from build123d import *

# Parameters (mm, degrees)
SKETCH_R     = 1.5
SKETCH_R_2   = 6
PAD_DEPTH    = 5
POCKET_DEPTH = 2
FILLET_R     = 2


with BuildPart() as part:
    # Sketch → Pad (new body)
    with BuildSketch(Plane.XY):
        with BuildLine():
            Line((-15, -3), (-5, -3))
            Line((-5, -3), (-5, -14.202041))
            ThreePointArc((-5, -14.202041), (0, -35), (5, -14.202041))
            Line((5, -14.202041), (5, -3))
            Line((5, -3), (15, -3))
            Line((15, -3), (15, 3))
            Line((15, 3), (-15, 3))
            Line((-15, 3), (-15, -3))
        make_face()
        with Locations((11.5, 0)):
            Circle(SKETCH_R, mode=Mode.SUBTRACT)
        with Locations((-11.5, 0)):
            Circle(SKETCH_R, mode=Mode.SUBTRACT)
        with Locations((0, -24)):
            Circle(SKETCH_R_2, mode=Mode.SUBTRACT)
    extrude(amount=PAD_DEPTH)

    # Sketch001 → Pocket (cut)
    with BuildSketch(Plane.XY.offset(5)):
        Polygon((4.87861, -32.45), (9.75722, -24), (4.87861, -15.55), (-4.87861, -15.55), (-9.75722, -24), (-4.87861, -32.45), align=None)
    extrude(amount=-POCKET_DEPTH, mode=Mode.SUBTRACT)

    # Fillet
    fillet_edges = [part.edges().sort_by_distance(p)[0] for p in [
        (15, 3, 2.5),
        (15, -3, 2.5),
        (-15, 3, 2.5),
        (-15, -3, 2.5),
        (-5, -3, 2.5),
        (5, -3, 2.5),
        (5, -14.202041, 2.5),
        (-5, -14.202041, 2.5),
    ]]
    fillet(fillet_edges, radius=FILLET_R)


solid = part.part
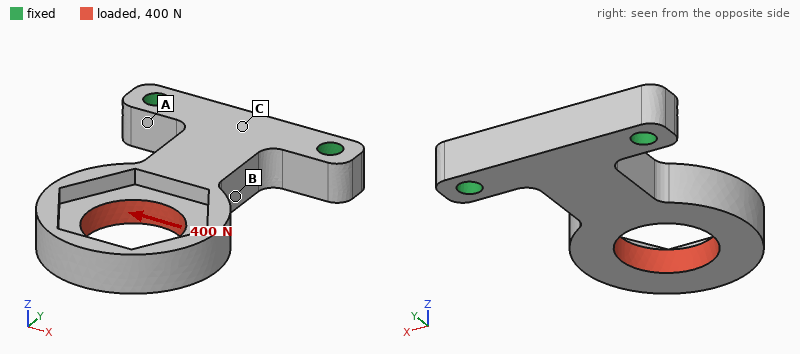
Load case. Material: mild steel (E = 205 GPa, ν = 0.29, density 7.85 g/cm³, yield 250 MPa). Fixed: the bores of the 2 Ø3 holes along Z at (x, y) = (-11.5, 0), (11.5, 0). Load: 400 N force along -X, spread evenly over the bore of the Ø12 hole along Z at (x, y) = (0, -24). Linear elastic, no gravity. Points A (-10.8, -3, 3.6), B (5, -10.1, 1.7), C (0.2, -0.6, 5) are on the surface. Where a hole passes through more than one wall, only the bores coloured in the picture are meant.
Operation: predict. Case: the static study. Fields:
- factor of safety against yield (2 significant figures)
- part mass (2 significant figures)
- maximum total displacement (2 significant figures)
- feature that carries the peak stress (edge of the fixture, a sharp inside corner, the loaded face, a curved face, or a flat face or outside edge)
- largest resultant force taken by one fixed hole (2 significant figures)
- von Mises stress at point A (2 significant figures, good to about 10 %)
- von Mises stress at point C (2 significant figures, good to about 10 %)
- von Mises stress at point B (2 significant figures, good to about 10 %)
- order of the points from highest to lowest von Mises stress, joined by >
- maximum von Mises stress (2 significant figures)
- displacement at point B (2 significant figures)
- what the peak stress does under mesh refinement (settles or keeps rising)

1.5
19 g
52 µm
a curved face
570 N
19 MPa
44 MPa
70 MPa
B > C > A
170 MPa
8.0 µm
settles
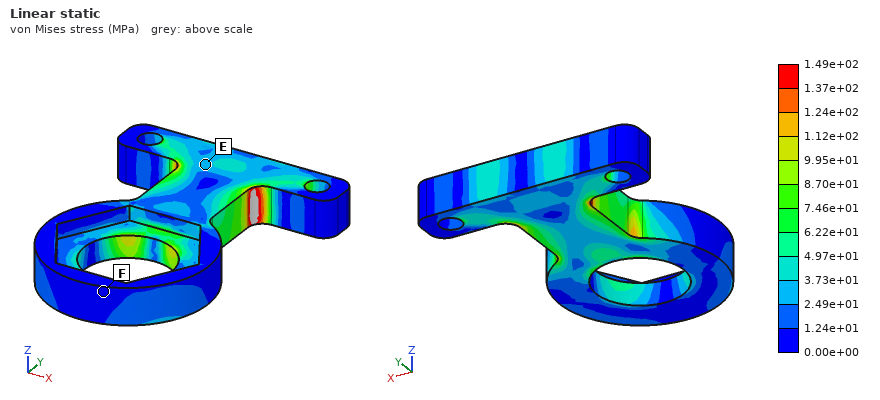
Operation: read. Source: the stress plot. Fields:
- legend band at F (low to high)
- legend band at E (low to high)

0.00e+00 to 1.24e+01 MPa
2.49e+01 to 3.73e+01 MPa
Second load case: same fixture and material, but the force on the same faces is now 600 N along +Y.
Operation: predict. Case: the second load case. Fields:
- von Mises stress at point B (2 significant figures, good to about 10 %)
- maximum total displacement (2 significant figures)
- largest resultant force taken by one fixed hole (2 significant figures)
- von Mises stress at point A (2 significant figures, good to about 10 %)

18 MPa
20 µm
320 N
19 MPa
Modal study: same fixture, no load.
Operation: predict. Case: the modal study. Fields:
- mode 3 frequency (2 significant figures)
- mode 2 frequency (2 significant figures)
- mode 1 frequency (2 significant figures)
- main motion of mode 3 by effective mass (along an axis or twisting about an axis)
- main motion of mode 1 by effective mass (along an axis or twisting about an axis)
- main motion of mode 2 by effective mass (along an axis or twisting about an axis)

8100 Hz
5400 Hz
2500 Hz
twisting about Y
along Z
along X
